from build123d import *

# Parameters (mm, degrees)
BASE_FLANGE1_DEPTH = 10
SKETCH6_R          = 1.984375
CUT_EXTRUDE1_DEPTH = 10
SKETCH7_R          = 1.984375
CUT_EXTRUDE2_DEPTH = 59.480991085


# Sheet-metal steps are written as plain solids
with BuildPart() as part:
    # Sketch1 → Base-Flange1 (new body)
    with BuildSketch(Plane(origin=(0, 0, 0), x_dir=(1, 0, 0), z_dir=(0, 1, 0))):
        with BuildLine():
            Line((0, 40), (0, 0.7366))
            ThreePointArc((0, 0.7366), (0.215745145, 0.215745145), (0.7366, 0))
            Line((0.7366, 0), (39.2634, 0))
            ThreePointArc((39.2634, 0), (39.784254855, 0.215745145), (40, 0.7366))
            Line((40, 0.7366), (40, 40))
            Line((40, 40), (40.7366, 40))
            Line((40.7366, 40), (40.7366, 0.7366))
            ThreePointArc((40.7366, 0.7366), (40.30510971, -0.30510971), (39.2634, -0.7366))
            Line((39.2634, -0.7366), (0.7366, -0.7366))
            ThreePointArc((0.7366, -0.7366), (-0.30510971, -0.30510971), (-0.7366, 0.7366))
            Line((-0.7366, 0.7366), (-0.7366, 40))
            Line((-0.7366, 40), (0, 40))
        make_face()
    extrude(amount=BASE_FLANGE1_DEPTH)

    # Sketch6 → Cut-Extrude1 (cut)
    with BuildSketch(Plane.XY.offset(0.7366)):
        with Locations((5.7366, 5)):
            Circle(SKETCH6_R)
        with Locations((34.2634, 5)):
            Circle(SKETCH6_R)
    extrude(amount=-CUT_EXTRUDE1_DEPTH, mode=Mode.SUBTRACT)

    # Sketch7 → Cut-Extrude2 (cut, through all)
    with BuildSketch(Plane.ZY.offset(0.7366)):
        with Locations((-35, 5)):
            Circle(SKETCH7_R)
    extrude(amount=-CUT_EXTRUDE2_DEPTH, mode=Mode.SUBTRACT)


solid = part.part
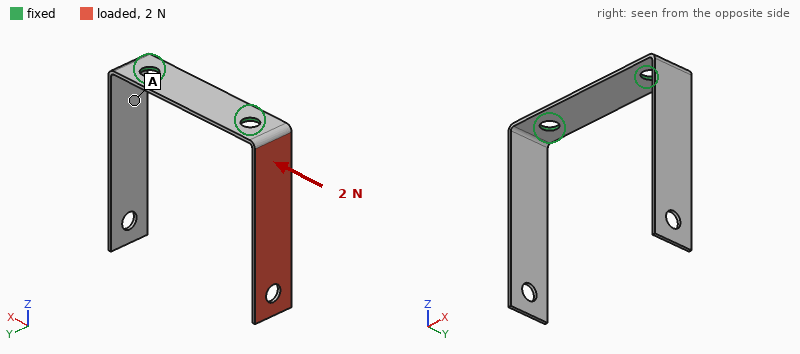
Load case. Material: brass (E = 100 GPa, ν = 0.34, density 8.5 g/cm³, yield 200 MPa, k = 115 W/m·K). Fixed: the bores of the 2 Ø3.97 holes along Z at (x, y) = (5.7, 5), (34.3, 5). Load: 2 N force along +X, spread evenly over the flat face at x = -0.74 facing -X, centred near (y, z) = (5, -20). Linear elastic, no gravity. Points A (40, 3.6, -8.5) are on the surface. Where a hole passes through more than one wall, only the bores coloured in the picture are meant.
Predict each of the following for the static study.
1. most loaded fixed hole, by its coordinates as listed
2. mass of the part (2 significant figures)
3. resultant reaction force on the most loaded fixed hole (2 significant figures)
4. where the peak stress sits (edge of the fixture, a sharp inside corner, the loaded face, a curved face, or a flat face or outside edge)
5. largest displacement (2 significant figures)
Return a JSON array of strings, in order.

["(5.7, 5)", "7.2 g", "2.0 N", "a flat face or outside edge", "0.66 mm"]
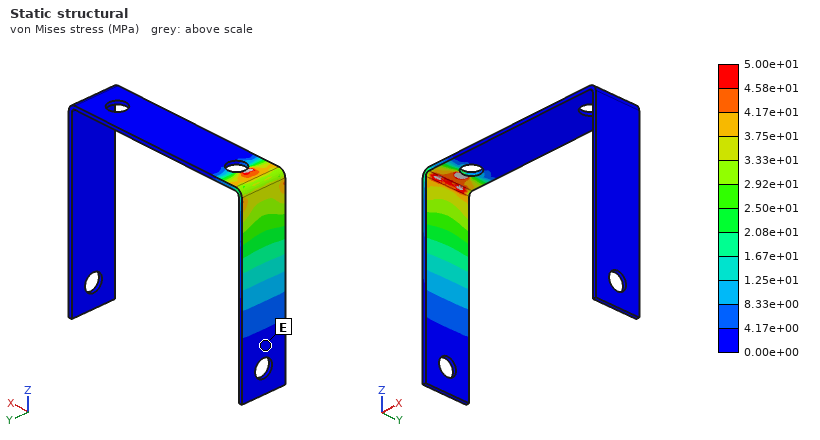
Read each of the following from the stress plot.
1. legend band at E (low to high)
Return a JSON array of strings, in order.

["0.00e+00 to 4.17e+00 MPa"]
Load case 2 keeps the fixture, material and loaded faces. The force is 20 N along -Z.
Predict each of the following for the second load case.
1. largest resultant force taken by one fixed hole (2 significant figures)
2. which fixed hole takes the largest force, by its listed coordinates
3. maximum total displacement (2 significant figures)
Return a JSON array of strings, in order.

["20 N", "(5.7, 5)", "0.40 mm"]
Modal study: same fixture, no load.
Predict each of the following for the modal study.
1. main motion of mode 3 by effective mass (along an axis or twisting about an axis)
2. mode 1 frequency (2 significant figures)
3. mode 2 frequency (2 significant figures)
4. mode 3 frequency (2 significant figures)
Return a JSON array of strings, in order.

["along Y", "220 Hz", "220 Hz", "580 Hz"]
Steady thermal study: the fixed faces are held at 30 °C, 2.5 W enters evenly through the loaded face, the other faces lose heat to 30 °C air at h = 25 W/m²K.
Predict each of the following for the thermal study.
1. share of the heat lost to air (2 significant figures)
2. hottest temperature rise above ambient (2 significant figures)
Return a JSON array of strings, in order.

["21 %", "57 K"]
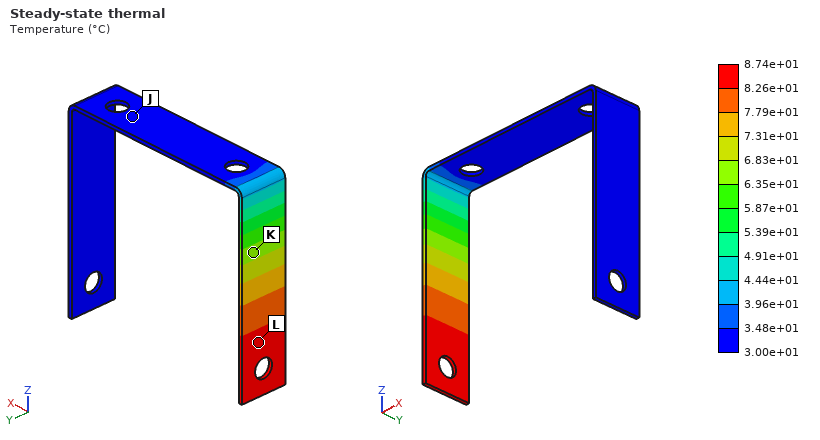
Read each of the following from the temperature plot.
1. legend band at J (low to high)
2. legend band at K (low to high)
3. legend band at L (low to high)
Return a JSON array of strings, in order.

["3.00e+01 to 3.48e+01 °C", "6.35e+01 to 6.83e+01 °C", "8.26e+01 to 8.74e+01 °C"]
